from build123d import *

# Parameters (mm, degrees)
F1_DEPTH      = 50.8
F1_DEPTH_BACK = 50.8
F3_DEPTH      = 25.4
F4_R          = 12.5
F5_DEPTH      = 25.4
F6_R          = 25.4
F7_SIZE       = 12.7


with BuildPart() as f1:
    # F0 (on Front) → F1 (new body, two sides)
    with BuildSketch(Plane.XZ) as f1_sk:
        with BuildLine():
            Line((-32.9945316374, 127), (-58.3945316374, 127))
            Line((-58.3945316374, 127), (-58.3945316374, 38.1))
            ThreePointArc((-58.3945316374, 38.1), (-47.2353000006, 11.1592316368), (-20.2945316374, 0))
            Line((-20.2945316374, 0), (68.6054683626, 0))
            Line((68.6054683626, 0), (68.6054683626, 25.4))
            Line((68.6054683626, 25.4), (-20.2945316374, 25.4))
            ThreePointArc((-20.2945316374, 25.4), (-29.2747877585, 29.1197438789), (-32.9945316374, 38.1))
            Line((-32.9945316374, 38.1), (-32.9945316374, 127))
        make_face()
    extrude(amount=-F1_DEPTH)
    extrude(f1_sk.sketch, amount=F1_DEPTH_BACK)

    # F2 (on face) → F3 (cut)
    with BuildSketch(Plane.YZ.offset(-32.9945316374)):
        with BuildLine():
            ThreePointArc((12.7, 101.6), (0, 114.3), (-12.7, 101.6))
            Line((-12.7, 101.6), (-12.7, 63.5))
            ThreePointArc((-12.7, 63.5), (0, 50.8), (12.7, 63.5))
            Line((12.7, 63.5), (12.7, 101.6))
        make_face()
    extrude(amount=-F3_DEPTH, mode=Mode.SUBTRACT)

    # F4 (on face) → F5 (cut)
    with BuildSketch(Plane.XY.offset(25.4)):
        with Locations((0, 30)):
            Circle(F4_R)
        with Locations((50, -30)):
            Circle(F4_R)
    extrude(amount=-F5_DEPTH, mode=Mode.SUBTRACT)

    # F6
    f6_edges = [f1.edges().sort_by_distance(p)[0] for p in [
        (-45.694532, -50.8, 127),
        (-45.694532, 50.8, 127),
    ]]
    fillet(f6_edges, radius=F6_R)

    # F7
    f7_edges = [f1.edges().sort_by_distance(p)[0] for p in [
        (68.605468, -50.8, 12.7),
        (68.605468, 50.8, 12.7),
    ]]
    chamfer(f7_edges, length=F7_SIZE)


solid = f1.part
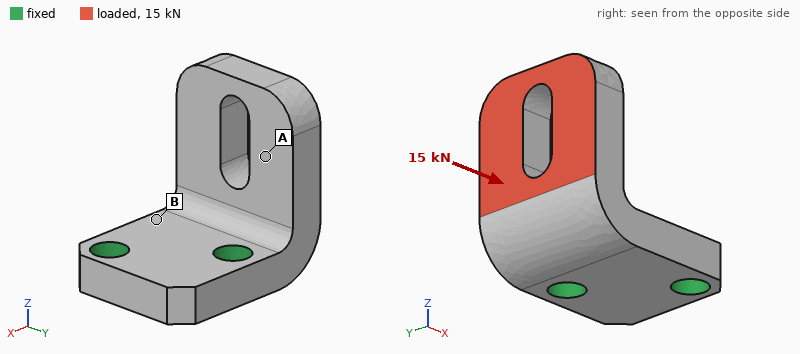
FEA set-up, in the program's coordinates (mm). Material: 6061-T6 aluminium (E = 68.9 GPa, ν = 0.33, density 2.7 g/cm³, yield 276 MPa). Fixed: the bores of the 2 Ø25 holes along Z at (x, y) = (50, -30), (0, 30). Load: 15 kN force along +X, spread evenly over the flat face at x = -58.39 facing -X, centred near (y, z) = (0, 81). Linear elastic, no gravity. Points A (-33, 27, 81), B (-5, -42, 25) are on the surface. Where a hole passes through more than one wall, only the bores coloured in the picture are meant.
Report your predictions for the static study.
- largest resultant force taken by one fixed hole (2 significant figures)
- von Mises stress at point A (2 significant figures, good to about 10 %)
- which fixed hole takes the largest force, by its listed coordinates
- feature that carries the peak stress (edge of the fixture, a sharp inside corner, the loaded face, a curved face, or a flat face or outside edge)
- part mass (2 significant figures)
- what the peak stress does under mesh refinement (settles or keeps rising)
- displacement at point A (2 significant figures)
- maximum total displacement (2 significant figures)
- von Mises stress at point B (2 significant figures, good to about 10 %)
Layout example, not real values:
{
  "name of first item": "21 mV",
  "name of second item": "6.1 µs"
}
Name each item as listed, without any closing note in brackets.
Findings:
{
  "largest resultant force taken by one fixed hole": "10 kN",
  "von Mises stress at point A": "23 MPa",
  "which fixed hole takes the largest force, by its listed coordinates": "(0, 30)",
  "feature that carries the peak stress": "edge of the fixture",
  "part mass": "1.3 kg",
  "what the peak stress does under mesh refinement": "keeps rising",
  "displacement at point A": "0.42 mm",
  "maximum total displacement": "0.85 mm",
  "von Mises stress at point B": "60 MPa"
}
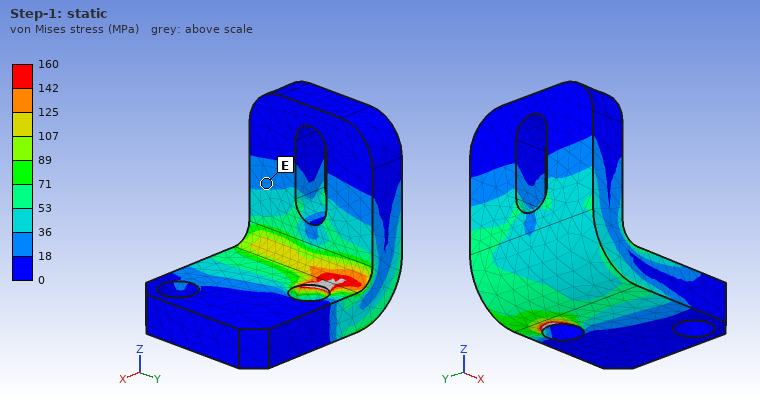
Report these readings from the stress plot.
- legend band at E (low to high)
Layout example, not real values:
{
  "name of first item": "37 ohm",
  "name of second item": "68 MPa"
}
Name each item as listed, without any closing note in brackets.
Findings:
{
  "legend band at E": "18 to 36 MPa"
}
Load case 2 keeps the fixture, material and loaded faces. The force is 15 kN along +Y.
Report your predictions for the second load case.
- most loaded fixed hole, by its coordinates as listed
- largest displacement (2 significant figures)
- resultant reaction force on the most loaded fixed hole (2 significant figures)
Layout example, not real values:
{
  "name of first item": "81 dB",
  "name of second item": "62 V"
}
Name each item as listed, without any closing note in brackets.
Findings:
{
  "most loaded fixed hole, by its coordinates as listed": "(0, 30)",
  "largest displacement": "0.37 mm",
  "resultant reaction force on the most loaded fixed hole": "19 kN"
}
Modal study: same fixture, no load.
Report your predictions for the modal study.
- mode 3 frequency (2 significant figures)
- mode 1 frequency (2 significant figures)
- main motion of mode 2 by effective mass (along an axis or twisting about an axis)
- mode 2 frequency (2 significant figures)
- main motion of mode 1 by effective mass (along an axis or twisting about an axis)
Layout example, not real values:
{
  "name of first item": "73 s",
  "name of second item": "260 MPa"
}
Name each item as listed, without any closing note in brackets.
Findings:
{
  "mode 3 frequency": "3200 Hz",
  "mode 1 frequency": "1100 Hz",
  "main motion of mode 2 by effective mass": "along Y",
  "mode 2 frequency": "1600 Hz",
  "main motion of mode 1 by effective mass": "along X"
}
